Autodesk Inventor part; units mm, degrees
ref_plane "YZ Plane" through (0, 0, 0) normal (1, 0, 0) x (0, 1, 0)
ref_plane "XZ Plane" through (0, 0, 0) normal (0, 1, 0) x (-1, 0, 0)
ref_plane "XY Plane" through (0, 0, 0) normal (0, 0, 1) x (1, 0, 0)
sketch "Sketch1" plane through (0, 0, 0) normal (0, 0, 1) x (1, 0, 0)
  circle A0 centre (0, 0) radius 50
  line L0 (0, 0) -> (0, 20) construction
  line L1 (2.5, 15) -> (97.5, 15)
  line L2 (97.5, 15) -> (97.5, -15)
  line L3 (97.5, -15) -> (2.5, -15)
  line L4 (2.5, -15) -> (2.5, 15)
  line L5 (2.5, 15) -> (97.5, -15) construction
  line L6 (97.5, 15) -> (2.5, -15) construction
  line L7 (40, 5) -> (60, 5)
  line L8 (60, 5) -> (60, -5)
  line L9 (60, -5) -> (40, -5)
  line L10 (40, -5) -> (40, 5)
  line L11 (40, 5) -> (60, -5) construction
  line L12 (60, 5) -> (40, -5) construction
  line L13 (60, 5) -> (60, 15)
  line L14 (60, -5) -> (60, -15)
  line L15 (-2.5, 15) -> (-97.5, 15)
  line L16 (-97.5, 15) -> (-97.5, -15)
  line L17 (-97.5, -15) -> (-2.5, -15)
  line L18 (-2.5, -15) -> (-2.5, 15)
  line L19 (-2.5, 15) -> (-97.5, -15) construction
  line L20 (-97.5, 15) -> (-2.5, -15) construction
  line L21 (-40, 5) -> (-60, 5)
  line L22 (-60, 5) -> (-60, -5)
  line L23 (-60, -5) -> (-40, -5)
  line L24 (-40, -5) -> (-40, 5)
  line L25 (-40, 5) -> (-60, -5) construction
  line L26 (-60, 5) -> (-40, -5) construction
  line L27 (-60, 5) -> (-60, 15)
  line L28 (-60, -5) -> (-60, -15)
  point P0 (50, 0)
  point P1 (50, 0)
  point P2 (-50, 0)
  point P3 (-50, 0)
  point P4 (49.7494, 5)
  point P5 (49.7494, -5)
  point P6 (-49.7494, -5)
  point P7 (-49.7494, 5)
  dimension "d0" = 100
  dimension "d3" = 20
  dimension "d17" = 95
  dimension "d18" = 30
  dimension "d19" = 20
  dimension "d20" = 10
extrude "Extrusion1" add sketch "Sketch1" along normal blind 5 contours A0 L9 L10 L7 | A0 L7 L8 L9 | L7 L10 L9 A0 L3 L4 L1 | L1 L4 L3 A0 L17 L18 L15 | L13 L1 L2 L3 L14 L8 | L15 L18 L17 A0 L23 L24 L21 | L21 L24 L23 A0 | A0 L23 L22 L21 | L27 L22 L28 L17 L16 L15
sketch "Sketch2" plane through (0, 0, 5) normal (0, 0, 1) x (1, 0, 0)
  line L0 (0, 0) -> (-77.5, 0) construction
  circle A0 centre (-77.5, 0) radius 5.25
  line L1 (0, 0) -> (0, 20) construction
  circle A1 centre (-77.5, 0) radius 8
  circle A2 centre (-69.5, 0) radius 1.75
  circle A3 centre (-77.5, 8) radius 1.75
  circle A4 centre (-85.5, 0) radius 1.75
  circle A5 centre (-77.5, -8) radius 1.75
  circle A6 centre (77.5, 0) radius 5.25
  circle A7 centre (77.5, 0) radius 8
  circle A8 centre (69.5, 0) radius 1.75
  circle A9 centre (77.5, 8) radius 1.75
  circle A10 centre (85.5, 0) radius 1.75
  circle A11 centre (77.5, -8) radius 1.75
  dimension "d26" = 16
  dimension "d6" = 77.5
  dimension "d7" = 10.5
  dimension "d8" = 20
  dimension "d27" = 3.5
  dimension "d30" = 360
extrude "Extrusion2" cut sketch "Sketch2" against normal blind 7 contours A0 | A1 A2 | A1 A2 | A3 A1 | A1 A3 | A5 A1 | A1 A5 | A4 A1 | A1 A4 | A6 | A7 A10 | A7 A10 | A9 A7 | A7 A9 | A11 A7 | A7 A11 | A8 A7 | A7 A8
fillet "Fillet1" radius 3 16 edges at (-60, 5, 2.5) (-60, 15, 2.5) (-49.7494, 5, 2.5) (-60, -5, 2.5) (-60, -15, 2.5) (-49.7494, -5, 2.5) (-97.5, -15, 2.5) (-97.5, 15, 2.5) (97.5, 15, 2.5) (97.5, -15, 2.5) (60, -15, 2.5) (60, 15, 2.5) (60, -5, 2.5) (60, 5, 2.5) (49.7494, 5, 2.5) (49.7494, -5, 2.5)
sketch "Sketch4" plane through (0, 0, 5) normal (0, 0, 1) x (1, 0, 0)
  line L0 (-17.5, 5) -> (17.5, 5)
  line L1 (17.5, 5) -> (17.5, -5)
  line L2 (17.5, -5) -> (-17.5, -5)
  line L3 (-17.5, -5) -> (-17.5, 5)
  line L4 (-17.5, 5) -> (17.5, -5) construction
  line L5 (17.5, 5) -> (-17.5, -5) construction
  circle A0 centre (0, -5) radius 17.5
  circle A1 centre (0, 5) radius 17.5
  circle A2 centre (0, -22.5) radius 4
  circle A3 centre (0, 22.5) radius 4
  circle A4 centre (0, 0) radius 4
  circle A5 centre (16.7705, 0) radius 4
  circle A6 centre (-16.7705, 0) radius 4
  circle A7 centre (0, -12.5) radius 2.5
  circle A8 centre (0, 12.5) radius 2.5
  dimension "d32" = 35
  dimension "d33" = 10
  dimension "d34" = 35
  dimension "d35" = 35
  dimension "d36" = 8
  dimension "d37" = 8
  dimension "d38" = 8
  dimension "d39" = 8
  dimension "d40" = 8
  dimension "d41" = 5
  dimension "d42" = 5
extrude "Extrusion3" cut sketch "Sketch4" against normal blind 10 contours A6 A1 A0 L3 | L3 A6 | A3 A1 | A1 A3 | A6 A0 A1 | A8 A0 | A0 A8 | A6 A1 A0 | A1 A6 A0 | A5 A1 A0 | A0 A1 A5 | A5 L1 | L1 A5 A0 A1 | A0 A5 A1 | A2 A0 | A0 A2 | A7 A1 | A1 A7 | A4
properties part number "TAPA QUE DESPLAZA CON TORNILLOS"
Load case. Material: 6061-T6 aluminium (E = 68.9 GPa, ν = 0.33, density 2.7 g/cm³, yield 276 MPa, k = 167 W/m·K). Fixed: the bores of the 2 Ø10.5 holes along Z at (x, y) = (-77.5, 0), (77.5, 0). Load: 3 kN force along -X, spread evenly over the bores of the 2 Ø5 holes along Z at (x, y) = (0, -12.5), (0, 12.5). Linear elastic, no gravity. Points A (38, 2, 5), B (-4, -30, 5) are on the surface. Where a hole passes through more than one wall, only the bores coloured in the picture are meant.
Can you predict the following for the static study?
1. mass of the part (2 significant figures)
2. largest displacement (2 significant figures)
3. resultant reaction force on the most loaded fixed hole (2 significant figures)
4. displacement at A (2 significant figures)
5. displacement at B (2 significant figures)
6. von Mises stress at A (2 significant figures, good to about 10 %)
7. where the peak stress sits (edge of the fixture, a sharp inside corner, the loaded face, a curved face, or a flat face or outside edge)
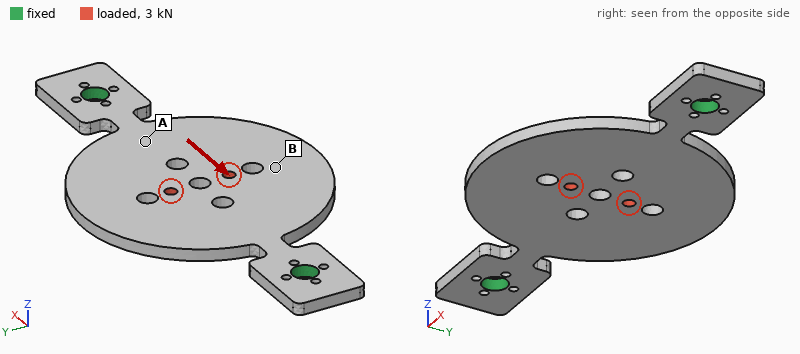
130 g
18 µm
1.5 kN
12 µm
15 µm
14 MPa
a curved face
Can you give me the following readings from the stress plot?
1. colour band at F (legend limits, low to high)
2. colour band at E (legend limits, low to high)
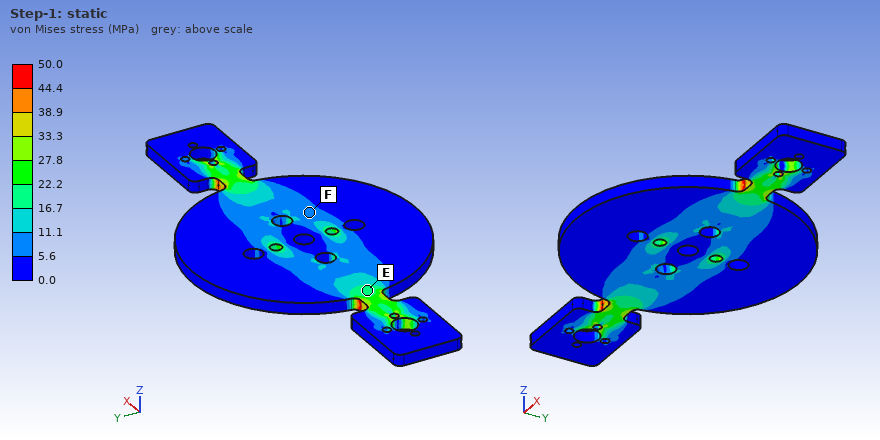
5.6 to 11.1 MPa
16.7 to 22.2 MPa
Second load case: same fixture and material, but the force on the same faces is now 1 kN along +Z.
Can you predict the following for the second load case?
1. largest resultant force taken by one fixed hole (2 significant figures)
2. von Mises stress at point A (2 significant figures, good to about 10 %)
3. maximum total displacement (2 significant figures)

500 N
39 MPa
0.65 mm
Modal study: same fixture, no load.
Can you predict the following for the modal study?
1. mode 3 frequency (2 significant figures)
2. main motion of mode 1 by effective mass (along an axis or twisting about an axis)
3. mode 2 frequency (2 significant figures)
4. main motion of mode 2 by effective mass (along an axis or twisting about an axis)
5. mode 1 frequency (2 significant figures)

2200 Hz
twisting about X
720 Hz
along Z
520 Hz
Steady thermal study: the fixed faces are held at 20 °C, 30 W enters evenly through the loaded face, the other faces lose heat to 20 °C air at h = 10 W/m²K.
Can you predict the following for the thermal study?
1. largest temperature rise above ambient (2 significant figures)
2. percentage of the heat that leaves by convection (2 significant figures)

46 K
22 %
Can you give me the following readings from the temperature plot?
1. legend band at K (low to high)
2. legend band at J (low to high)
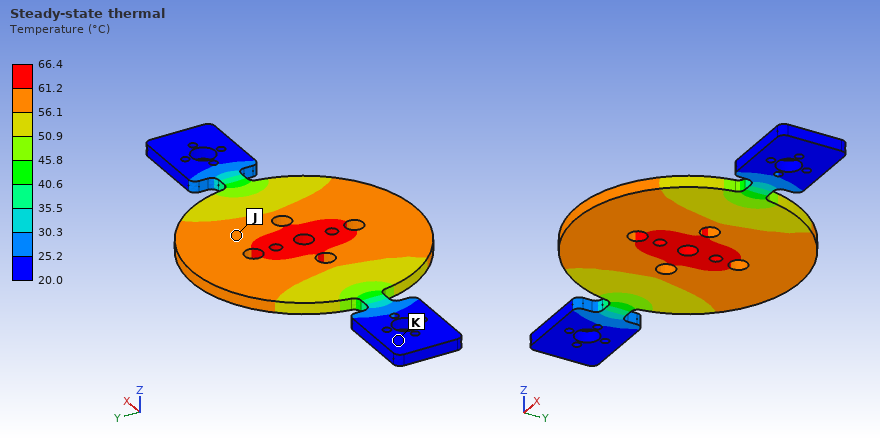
20.0 to 25.2 °C
56.1 to 61.2 °C
